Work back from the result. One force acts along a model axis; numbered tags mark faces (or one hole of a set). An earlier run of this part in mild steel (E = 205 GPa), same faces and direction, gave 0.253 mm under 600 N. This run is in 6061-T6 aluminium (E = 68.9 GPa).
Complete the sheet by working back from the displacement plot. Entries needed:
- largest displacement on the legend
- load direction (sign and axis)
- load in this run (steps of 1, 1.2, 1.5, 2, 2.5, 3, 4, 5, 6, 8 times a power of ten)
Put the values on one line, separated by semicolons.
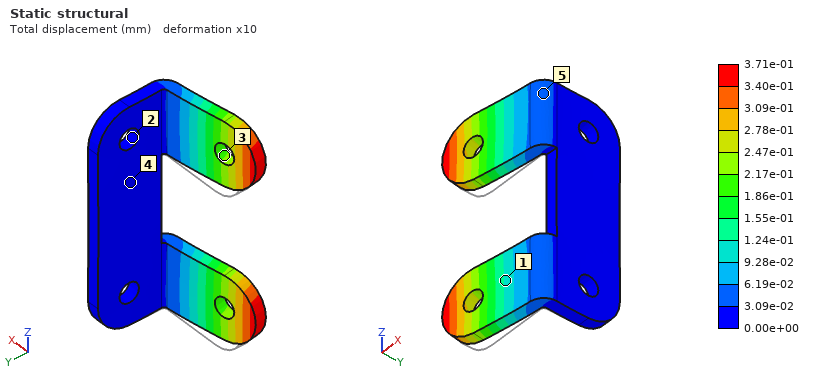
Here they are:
3.71e-01 mm; -Y; 300 N
